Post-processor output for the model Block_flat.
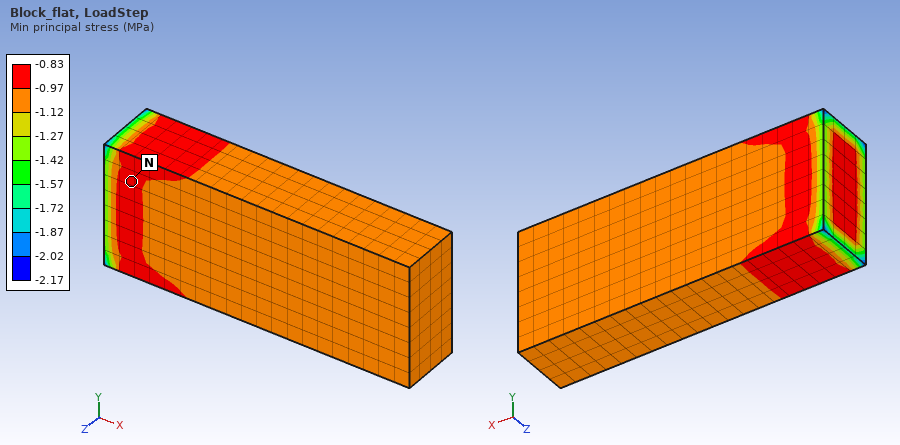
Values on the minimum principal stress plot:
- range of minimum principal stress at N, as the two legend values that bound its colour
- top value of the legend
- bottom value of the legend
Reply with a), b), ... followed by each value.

a) -0.97 to -0.83 MPa
b) -0.83 MPa
c) -2.17 MPa
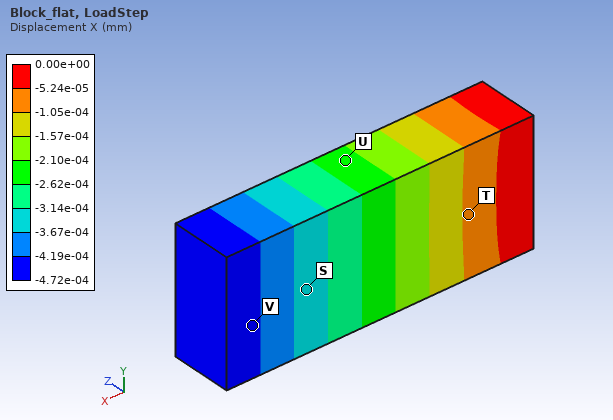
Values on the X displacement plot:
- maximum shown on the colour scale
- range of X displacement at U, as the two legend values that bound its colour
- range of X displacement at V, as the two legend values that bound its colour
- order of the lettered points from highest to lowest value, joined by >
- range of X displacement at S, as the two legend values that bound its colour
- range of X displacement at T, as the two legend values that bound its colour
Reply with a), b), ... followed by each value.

a) 0.00e+00 mm
b) -2.62e-04 to -2.10e-04 mm
c) -4.72e-04 to -4.19e-04 mm
d) T > U > S > V
e) -3.67e-04 to -3.14e-04 mm
f) -1.05e-04 to -5.24e-05 mm
